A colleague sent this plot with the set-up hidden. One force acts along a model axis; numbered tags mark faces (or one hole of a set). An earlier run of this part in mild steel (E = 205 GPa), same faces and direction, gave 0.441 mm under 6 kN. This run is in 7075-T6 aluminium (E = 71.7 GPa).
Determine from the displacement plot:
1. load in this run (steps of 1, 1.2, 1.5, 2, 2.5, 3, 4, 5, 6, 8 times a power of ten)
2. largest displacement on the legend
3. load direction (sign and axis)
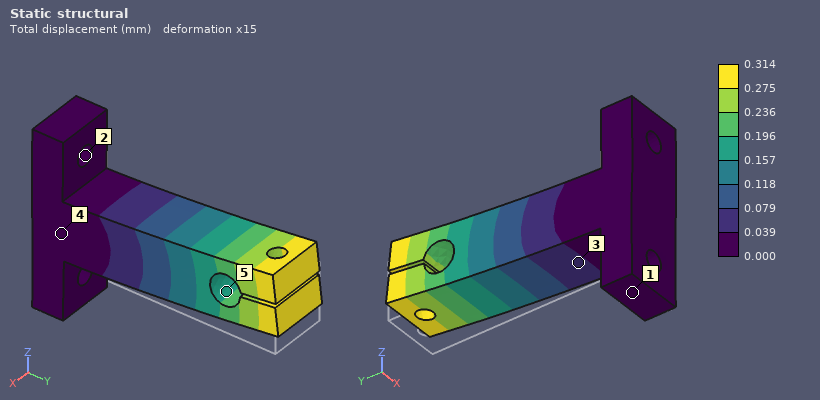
1.5 kN
0.314 mm
+Z
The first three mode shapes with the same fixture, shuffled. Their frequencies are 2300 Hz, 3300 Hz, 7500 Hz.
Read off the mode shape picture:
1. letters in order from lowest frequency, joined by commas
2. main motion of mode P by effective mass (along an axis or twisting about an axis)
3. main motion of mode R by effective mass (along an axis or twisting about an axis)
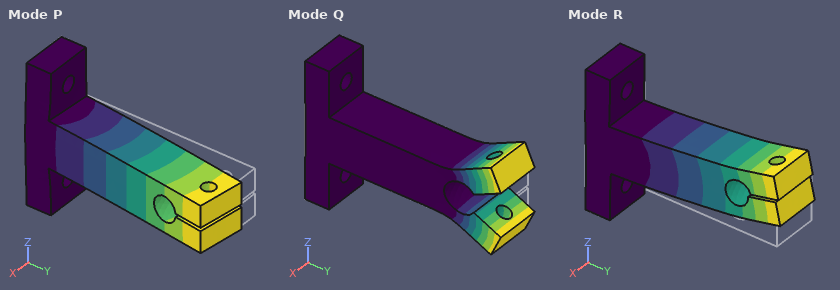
P, R, Q
along X
along Z
